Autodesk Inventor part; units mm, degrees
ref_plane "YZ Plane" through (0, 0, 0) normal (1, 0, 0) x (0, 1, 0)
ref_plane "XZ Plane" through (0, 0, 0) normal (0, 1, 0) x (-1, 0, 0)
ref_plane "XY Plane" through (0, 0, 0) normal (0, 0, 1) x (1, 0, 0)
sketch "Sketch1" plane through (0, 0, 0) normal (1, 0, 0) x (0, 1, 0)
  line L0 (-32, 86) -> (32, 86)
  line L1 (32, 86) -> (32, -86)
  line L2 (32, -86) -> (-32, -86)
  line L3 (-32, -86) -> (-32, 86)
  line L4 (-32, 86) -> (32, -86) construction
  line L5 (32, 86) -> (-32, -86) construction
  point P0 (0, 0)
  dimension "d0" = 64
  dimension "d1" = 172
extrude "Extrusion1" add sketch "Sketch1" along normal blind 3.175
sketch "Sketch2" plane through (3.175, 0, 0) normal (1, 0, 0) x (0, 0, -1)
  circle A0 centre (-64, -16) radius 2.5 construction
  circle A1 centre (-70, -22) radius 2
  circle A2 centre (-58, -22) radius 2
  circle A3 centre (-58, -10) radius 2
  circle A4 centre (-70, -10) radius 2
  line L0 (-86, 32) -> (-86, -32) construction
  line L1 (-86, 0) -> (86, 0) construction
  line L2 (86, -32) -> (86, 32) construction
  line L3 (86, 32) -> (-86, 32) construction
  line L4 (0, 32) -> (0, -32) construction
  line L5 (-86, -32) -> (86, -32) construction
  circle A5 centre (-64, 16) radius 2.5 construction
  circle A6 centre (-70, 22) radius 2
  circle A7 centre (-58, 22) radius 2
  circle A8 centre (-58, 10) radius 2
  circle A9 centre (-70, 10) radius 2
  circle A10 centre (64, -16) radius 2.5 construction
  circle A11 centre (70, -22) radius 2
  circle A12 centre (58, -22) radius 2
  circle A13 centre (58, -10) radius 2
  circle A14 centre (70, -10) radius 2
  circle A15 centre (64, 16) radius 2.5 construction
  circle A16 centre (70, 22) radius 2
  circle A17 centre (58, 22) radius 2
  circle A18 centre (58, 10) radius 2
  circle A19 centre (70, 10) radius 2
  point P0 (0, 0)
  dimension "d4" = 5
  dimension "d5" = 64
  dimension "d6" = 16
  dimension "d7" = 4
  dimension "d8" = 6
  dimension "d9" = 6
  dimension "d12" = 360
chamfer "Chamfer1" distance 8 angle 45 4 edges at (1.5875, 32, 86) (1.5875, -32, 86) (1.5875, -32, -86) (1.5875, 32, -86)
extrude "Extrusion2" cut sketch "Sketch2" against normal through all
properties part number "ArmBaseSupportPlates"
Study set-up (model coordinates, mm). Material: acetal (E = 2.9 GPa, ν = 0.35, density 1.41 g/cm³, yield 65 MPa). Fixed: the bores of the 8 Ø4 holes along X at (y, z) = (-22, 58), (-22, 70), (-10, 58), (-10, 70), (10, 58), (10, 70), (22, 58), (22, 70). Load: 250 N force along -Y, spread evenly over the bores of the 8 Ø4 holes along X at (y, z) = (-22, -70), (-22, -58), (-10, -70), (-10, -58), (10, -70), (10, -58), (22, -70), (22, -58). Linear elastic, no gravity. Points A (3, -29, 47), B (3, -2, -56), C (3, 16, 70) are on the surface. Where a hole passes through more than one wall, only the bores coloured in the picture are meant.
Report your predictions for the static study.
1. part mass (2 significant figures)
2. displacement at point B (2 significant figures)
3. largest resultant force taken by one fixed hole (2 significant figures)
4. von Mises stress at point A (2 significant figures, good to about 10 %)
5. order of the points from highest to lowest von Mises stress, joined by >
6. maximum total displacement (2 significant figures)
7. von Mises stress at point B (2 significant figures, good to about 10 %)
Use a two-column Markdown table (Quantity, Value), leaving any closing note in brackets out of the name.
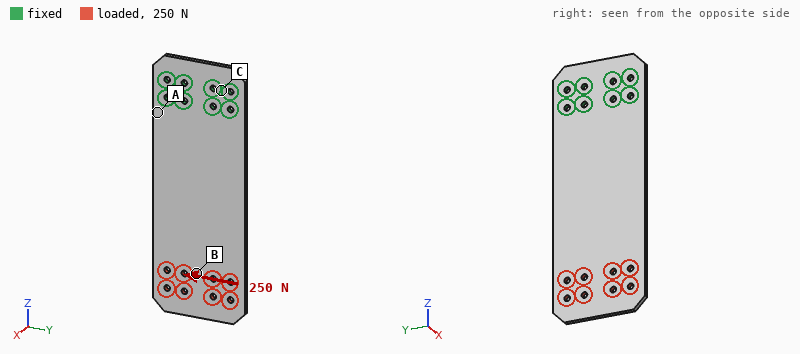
| Quantity | Value |
|---|---|
| part mass | 48 g |
| displacement at point B | 0.89 mm |
| largest resultant force taken by one fixed hole | 460 N |
| von Mises stress at point A | 10 MPa |
| order of the points from highest to lowest von Mises stress, joined by > | A > B > C |
| maximum total displacement | 1.2 mm |
| von Mises stress at point B | 2.9 MPa |
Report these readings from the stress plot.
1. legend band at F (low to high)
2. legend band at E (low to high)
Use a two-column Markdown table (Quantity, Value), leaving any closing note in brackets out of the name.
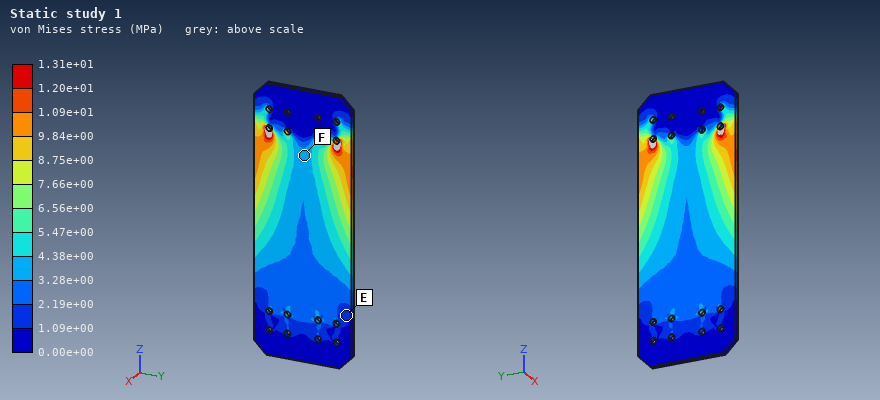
| Quantity | Value |
|---|---|
| legend band at F | 3.28e+00 to 4.38e+00 MPa |
| legend band at E | 1.09e+00 to 2.19e+00 MPa |
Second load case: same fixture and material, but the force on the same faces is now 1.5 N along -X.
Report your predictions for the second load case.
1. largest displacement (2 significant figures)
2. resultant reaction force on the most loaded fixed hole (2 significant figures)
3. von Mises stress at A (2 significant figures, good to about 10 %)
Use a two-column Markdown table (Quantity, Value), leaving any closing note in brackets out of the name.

| Quantity | Value |
|---|---|
| largest displacement | 2.2 mm |
| resultant reaction force on the most loaded fixed hole | 2.4 N |
| von Mises stress at A | 1.5 MPa |
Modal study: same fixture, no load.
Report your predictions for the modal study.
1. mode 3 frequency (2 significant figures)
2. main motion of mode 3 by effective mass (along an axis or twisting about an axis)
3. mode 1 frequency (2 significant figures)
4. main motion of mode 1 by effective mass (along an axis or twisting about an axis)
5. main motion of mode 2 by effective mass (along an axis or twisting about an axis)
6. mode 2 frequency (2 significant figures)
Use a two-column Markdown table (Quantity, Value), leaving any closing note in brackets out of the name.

| Quantity | Value |
|---|---|
| mode 3 frequency | 230 Hz |
| main motion of mode 3 by effective mass | along X |
| mode 1 frequency | 38 Hz |
| main motion of mode 1 by effective mass | along X |
| main motion of mode 2 by effective mass | twisting about Z |
| mode 2 frequency | 170 Hz |
